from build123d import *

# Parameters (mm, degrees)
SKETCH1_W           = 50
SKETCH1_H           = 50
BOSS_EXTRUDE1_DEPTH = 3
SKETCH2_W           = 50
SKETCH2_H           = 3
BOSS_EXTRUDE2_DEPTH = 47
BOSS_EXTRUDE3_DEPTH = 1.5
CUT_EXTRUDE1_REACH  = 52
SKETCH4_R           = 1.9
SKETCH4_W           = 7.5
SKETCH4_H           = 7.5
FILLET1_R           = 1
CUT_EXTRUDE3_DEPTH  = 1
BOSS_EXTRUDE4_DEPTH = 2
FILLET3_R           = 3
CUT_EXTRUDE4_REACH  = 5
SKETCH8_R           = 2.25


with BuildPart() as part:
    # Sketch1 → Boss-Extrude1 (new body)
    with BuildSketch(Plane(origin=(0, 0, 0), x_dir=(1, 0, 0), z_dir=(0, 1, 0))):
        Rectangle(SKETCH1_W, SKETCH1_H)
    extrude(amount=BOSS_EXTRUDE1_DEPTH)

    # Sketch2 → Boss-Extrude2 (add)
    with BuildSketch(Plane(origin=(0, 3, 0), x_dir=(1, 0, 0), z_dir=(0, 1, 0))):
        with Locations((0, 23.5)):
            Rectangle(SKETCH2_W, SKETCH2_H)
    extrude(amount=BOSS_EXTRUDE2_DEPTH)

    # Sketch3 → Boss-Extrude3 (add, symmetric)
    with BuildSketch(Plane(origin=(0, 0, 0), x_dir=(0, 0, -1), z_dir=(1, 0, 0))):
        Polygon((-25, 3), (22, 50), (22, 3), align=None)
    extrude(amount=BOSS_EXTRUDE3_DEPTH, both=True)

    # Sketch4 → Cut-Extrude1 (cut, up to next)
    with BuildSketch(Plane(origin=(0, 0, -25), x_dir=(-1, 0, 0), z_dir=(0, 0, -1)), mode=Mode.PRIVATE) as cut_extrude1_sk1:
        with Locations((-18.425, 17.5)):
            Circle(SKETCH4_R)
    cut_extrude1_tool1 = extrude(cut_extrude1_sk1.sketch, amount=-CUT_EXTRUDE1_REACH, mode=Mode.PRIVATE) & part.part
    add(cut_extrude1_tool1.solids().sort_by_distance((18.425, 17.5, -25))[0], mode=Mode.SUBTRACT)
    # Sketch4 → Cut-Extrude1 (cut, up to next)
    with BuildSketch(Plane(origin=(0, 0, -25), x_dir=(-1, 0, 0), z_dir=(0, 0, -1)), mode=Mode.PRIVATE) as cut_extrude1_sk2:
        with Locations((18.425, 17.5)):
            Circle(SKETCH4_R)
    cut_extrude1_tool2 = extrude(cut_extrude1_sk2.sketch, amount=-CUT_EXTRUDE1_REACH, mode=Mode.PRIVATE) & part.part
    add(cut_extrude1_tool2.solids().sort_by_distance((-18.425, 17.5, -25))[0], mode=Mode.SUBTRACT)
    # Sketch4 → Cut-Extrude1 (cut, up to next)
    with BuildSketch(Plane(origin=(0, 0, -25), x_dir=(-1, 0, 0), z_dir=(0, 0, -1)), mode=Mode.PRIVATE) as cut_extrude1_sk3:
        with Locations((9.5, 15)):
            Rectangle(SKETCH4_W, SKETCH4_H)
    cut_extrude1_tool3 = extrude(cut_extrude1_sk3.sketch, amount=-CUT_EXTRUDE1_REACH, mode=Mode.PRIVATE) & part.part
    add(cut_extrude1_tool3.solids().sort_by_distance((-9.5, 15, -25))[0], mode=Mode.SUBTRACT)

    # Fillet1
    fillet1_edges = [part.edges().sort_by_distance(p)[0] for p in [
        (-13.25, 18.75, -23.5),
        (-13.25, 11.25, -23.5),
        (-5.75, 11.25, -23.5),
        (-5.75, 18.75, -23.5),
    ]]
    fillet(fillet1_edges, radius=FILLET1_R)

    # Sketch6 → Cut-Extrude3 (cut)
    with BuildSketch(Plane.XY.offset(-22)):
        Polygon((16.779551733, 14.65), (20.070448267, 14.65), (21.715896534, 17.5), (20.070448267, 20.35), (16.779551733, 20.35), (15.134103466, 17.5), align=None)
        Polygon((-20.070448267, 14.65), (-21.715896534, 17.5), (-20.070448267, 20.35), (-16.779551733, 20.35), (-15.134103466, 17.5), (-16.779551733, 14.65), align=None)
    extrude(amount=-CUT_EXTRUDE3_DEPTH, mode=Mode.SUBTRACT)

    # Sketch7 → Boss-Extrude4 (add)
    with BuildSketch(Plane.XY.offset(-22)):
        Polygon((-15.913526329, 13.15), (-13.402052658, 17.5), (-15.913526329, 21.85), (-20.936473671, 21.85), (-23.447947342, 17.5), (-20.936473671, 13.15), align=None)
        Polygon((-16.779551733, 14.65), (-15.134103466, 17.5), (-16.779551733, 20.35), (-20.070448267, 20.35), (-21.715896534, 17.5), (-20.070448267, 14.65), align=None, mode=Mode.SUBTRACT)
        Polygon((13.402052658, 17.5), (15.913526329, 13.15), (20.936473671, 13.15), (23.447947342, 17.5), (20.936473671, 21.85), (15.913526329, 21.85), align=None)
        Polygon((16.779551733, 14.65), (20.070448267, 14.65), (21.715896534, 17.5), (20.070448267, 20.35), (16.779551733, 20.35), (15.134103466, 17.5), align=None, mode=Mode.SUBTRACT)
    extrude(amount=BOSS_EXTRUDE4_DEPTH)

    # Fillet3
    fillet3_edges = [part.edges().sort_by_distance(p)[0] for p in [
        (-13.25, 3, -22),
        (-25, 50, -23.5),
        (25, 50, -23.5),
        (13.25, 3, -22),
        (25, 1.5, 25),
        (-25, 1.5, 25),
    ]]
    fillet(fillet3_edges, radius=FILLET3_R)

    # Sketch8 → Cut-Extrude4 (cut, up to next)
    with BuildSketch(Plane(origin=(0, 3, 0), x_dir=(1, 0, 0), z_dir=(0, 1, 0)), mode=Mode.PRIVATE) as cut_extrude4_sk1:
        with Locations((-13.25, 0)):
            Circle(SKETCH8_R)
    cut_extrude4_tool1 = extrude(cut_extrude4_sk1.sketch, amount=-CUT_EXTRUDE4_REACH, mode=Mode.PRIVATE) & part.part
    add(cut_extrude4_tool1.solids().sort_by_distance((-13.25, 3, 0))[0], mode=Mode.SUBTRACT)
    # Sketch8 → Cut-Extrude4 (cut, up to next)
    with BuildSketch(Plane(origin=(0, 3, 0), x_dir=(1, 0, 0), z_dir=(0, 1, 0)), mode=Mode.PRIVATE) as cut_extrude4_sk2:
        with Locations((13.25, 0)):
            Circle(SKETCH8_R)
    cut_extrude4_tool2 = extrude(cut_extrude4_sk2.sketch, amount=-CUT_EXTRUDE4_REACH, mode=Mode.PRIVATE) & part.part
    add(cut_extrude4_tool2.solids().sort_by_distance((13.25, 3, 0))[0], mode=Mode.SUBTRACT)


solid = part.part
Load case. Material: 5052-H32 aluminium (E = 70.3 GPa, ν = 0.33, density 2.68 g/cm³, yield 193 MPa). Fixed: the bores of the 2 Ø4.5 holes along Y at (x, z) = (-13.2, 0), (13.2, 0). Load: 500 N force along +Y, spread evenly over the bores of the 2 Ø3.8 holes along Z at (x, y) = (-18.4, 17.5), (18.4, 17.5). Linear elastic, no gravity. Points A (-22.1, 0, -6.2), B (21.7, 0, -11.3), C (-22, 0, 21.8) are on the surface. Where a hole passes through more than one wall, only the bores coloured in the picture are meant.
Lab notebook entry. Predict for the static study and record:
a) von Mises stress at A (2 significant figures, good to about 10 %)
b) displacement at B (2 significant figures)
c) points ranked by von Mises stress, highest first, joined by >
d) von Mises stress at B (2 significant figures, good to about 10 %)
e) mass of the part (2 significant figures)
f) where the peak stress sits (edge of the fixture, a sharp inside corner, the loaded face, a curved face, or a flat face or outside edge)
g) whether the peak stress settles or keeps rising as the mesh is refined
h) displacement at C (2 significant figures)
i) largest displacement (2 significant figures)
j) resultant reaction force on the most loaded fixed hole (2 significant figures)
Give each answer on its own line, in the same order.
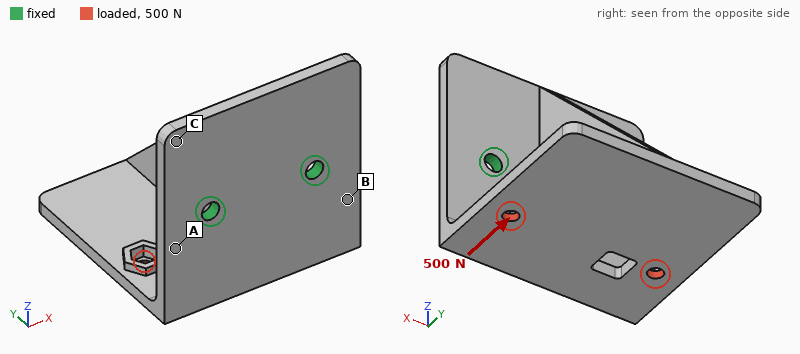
50 MPa
0.047 mm
A > B > C
29 MPa
47 g
edge of the fixture
keeps rising
0.070 mm
0.29 mm
260 N
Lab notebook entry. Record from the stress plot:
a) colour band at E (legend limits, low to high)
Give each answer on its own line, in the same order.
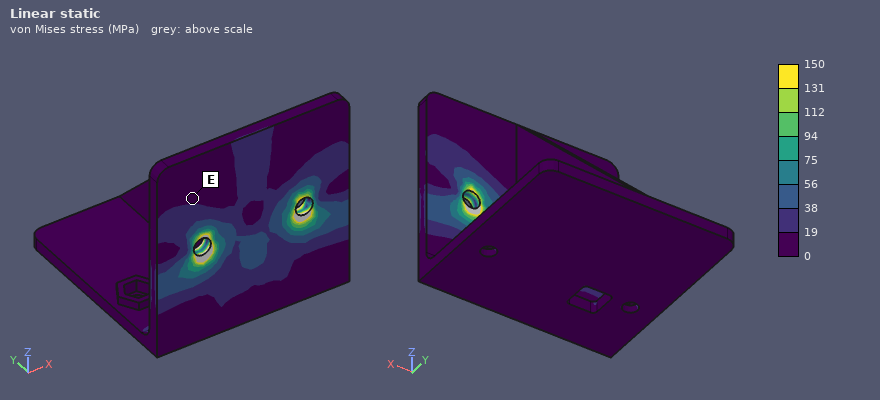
0 to 19 MPa
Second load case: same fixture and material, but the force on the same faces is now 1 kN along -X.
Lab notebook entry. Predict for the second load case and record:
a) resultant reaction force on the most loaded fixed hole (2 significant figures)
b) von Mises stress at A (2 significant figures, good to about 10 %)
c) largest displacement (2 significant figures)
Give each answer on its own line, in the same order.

1.1 kN
72 MPa
0.43 mm
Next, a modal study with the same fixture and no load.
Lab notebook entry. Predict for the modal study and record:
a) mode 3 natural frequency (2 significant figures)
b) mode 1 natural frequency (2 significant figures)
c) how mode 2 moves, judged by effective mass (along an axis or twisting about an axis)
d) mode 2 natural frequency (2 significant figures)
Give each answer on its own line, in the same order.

2800 Hz
1300 Hz
along X
1500 Hz
